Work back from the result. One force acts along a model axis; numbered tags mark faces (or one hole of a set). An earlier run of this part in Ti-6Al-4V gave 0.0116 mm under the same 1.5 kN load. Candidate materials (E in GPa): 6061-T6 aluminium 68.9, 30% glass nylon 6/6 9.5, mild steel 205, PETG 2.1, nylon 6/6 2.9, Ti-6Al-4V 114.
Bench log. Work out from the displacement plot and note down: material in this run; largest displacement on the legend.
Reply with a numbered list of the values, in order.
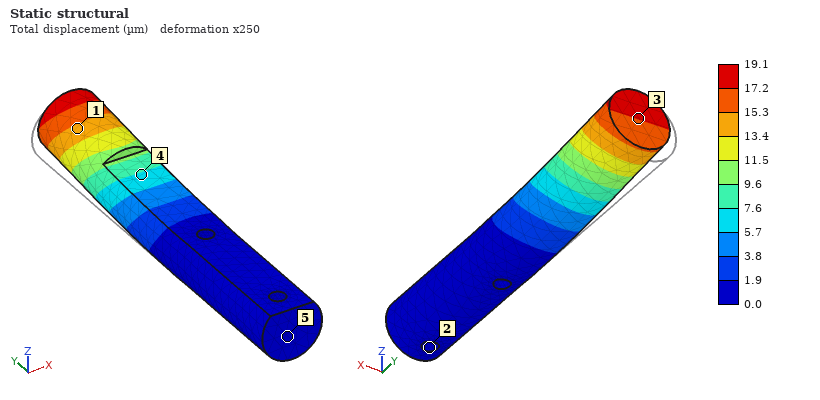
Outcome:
1. 6061-T6 aluminium
2. 19.1 µm
